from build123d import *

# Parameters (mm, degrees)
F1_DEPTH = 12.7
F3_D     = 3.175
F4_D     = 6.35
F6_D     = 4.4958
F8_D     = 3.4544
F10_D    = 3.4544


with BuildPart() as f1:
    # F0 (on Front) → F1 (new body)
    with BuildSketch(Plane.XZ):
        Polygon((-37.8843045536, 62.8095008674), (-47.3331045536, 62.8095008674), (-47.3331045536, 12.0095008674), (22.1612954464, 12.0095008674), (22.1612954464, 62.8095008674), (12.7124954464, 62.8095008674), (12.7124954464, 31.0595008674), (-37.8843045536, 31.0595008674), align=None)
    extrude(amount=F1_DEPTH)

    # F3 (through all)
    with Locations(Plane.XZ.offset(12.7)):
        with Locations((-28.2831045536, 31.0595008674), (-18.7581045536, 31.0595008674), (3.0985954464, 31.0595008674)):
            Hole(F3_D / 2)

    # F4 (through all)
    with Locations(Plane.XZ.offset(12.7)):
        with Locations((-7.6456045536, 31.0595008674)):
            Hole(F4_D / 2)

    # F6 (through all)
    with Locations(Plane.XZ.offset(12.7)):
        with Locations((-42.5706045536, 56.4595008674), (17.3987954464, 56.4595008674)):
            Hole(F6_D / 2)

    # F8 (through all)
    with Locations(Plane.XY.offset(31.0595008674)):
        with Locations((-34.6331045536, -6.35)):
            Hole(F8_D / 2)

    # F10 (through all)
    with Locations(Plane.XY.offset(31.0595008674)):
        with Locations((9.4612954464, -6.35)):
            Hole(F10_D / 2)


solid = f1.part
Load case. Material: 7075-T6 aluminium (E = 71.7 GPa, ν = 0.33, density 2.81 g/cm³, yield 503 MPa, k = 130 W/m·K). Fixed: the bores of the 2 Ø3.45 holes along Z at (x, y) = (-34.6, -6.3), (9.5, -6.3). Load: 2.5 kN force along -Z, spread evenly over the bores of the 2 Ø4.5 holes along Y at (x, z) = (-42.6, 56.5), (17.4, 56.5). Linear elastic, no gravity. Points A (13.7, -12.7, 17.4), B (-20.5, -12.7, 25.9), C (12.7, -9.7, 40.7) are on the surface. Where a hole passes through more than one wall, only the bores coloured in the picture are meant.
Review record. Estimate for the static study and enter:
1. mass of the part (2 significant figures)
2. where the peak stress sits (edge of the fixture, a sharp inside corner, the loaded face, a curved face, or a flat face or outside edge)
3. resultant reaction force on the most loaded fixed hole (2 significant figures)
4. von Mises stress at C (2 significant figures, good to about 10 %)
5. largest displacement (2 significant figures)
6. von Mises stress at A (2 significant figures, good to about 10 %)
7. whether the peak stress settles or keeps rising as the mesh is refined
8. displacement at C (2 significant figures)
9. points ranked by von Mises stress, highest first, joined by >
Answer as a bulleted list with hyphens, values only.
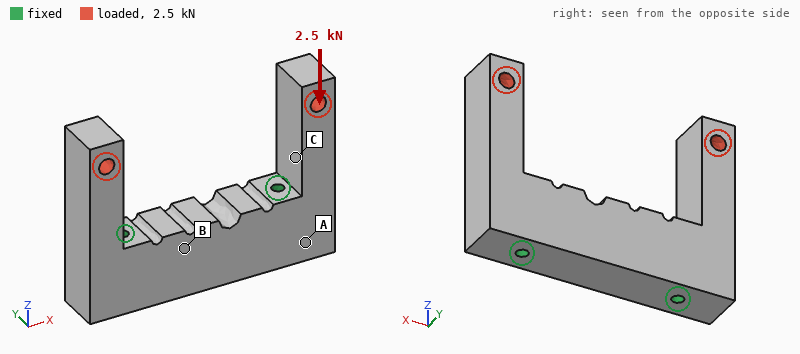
- 66 g
- edge of the fixture
- 1.3 kN
- 11 MPa
- 12 µm
- 6.4 MPa
- keeps rising
- 4.7 µm
- C > A > B
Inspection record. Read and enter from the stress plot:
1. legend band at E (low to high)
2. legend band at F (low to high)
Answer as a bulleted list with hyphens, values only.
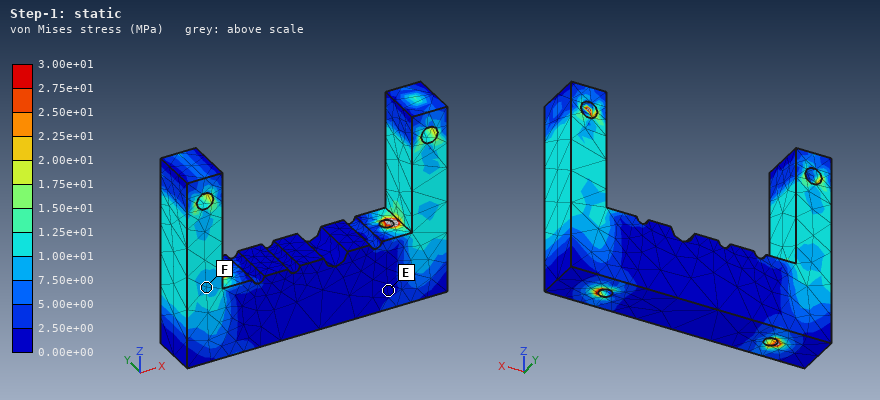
- 0.00e+00 to 2.50e+00 MPa
- 7.50e+00 to 1.00e+01 MPa
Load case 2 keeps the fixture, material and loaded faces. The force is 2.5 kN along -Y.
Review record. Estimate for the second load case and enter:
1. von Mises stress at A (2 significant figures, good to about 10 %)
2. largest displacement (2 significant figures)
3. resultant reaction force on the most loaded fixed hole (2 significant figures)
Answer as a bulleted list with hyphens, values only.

- 39 MPa
- 0.21 mm
- 1.3 kN
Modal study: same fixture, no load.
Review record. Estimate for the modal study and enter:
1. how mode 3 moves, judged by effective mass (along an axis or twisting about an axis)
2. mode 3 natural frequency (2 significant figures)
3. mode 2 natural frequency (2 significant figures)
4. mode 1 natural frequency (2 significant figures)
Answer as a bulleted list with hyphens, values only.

- along Y
- 6200 Hz
- 5600 Hz
- 5600 Hz
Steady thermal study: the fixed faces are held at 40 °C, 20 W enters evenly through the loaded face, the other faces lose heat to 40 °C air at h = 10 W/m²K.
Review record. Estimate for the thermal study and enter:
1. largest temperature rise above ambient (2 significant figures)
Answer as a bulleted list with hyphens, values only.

- 22 K
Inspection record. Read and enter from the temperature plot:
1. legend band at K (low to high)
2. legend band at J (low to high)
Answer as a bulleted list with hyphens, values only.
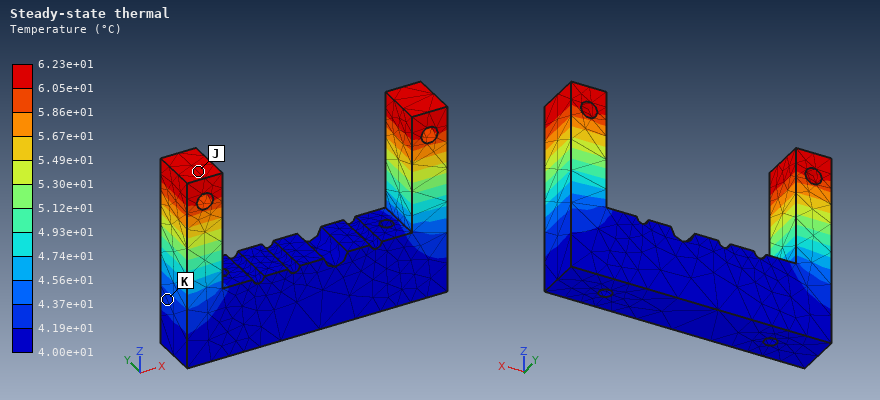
- 4.19e+01 to 4.37e+01 °C
- 6.05e+01 to 6.23e+01 °C
